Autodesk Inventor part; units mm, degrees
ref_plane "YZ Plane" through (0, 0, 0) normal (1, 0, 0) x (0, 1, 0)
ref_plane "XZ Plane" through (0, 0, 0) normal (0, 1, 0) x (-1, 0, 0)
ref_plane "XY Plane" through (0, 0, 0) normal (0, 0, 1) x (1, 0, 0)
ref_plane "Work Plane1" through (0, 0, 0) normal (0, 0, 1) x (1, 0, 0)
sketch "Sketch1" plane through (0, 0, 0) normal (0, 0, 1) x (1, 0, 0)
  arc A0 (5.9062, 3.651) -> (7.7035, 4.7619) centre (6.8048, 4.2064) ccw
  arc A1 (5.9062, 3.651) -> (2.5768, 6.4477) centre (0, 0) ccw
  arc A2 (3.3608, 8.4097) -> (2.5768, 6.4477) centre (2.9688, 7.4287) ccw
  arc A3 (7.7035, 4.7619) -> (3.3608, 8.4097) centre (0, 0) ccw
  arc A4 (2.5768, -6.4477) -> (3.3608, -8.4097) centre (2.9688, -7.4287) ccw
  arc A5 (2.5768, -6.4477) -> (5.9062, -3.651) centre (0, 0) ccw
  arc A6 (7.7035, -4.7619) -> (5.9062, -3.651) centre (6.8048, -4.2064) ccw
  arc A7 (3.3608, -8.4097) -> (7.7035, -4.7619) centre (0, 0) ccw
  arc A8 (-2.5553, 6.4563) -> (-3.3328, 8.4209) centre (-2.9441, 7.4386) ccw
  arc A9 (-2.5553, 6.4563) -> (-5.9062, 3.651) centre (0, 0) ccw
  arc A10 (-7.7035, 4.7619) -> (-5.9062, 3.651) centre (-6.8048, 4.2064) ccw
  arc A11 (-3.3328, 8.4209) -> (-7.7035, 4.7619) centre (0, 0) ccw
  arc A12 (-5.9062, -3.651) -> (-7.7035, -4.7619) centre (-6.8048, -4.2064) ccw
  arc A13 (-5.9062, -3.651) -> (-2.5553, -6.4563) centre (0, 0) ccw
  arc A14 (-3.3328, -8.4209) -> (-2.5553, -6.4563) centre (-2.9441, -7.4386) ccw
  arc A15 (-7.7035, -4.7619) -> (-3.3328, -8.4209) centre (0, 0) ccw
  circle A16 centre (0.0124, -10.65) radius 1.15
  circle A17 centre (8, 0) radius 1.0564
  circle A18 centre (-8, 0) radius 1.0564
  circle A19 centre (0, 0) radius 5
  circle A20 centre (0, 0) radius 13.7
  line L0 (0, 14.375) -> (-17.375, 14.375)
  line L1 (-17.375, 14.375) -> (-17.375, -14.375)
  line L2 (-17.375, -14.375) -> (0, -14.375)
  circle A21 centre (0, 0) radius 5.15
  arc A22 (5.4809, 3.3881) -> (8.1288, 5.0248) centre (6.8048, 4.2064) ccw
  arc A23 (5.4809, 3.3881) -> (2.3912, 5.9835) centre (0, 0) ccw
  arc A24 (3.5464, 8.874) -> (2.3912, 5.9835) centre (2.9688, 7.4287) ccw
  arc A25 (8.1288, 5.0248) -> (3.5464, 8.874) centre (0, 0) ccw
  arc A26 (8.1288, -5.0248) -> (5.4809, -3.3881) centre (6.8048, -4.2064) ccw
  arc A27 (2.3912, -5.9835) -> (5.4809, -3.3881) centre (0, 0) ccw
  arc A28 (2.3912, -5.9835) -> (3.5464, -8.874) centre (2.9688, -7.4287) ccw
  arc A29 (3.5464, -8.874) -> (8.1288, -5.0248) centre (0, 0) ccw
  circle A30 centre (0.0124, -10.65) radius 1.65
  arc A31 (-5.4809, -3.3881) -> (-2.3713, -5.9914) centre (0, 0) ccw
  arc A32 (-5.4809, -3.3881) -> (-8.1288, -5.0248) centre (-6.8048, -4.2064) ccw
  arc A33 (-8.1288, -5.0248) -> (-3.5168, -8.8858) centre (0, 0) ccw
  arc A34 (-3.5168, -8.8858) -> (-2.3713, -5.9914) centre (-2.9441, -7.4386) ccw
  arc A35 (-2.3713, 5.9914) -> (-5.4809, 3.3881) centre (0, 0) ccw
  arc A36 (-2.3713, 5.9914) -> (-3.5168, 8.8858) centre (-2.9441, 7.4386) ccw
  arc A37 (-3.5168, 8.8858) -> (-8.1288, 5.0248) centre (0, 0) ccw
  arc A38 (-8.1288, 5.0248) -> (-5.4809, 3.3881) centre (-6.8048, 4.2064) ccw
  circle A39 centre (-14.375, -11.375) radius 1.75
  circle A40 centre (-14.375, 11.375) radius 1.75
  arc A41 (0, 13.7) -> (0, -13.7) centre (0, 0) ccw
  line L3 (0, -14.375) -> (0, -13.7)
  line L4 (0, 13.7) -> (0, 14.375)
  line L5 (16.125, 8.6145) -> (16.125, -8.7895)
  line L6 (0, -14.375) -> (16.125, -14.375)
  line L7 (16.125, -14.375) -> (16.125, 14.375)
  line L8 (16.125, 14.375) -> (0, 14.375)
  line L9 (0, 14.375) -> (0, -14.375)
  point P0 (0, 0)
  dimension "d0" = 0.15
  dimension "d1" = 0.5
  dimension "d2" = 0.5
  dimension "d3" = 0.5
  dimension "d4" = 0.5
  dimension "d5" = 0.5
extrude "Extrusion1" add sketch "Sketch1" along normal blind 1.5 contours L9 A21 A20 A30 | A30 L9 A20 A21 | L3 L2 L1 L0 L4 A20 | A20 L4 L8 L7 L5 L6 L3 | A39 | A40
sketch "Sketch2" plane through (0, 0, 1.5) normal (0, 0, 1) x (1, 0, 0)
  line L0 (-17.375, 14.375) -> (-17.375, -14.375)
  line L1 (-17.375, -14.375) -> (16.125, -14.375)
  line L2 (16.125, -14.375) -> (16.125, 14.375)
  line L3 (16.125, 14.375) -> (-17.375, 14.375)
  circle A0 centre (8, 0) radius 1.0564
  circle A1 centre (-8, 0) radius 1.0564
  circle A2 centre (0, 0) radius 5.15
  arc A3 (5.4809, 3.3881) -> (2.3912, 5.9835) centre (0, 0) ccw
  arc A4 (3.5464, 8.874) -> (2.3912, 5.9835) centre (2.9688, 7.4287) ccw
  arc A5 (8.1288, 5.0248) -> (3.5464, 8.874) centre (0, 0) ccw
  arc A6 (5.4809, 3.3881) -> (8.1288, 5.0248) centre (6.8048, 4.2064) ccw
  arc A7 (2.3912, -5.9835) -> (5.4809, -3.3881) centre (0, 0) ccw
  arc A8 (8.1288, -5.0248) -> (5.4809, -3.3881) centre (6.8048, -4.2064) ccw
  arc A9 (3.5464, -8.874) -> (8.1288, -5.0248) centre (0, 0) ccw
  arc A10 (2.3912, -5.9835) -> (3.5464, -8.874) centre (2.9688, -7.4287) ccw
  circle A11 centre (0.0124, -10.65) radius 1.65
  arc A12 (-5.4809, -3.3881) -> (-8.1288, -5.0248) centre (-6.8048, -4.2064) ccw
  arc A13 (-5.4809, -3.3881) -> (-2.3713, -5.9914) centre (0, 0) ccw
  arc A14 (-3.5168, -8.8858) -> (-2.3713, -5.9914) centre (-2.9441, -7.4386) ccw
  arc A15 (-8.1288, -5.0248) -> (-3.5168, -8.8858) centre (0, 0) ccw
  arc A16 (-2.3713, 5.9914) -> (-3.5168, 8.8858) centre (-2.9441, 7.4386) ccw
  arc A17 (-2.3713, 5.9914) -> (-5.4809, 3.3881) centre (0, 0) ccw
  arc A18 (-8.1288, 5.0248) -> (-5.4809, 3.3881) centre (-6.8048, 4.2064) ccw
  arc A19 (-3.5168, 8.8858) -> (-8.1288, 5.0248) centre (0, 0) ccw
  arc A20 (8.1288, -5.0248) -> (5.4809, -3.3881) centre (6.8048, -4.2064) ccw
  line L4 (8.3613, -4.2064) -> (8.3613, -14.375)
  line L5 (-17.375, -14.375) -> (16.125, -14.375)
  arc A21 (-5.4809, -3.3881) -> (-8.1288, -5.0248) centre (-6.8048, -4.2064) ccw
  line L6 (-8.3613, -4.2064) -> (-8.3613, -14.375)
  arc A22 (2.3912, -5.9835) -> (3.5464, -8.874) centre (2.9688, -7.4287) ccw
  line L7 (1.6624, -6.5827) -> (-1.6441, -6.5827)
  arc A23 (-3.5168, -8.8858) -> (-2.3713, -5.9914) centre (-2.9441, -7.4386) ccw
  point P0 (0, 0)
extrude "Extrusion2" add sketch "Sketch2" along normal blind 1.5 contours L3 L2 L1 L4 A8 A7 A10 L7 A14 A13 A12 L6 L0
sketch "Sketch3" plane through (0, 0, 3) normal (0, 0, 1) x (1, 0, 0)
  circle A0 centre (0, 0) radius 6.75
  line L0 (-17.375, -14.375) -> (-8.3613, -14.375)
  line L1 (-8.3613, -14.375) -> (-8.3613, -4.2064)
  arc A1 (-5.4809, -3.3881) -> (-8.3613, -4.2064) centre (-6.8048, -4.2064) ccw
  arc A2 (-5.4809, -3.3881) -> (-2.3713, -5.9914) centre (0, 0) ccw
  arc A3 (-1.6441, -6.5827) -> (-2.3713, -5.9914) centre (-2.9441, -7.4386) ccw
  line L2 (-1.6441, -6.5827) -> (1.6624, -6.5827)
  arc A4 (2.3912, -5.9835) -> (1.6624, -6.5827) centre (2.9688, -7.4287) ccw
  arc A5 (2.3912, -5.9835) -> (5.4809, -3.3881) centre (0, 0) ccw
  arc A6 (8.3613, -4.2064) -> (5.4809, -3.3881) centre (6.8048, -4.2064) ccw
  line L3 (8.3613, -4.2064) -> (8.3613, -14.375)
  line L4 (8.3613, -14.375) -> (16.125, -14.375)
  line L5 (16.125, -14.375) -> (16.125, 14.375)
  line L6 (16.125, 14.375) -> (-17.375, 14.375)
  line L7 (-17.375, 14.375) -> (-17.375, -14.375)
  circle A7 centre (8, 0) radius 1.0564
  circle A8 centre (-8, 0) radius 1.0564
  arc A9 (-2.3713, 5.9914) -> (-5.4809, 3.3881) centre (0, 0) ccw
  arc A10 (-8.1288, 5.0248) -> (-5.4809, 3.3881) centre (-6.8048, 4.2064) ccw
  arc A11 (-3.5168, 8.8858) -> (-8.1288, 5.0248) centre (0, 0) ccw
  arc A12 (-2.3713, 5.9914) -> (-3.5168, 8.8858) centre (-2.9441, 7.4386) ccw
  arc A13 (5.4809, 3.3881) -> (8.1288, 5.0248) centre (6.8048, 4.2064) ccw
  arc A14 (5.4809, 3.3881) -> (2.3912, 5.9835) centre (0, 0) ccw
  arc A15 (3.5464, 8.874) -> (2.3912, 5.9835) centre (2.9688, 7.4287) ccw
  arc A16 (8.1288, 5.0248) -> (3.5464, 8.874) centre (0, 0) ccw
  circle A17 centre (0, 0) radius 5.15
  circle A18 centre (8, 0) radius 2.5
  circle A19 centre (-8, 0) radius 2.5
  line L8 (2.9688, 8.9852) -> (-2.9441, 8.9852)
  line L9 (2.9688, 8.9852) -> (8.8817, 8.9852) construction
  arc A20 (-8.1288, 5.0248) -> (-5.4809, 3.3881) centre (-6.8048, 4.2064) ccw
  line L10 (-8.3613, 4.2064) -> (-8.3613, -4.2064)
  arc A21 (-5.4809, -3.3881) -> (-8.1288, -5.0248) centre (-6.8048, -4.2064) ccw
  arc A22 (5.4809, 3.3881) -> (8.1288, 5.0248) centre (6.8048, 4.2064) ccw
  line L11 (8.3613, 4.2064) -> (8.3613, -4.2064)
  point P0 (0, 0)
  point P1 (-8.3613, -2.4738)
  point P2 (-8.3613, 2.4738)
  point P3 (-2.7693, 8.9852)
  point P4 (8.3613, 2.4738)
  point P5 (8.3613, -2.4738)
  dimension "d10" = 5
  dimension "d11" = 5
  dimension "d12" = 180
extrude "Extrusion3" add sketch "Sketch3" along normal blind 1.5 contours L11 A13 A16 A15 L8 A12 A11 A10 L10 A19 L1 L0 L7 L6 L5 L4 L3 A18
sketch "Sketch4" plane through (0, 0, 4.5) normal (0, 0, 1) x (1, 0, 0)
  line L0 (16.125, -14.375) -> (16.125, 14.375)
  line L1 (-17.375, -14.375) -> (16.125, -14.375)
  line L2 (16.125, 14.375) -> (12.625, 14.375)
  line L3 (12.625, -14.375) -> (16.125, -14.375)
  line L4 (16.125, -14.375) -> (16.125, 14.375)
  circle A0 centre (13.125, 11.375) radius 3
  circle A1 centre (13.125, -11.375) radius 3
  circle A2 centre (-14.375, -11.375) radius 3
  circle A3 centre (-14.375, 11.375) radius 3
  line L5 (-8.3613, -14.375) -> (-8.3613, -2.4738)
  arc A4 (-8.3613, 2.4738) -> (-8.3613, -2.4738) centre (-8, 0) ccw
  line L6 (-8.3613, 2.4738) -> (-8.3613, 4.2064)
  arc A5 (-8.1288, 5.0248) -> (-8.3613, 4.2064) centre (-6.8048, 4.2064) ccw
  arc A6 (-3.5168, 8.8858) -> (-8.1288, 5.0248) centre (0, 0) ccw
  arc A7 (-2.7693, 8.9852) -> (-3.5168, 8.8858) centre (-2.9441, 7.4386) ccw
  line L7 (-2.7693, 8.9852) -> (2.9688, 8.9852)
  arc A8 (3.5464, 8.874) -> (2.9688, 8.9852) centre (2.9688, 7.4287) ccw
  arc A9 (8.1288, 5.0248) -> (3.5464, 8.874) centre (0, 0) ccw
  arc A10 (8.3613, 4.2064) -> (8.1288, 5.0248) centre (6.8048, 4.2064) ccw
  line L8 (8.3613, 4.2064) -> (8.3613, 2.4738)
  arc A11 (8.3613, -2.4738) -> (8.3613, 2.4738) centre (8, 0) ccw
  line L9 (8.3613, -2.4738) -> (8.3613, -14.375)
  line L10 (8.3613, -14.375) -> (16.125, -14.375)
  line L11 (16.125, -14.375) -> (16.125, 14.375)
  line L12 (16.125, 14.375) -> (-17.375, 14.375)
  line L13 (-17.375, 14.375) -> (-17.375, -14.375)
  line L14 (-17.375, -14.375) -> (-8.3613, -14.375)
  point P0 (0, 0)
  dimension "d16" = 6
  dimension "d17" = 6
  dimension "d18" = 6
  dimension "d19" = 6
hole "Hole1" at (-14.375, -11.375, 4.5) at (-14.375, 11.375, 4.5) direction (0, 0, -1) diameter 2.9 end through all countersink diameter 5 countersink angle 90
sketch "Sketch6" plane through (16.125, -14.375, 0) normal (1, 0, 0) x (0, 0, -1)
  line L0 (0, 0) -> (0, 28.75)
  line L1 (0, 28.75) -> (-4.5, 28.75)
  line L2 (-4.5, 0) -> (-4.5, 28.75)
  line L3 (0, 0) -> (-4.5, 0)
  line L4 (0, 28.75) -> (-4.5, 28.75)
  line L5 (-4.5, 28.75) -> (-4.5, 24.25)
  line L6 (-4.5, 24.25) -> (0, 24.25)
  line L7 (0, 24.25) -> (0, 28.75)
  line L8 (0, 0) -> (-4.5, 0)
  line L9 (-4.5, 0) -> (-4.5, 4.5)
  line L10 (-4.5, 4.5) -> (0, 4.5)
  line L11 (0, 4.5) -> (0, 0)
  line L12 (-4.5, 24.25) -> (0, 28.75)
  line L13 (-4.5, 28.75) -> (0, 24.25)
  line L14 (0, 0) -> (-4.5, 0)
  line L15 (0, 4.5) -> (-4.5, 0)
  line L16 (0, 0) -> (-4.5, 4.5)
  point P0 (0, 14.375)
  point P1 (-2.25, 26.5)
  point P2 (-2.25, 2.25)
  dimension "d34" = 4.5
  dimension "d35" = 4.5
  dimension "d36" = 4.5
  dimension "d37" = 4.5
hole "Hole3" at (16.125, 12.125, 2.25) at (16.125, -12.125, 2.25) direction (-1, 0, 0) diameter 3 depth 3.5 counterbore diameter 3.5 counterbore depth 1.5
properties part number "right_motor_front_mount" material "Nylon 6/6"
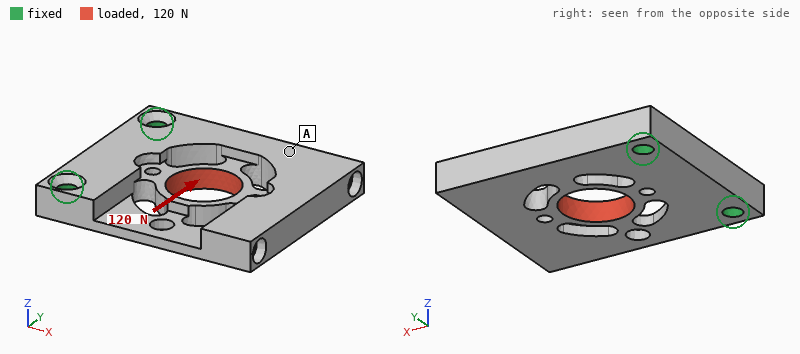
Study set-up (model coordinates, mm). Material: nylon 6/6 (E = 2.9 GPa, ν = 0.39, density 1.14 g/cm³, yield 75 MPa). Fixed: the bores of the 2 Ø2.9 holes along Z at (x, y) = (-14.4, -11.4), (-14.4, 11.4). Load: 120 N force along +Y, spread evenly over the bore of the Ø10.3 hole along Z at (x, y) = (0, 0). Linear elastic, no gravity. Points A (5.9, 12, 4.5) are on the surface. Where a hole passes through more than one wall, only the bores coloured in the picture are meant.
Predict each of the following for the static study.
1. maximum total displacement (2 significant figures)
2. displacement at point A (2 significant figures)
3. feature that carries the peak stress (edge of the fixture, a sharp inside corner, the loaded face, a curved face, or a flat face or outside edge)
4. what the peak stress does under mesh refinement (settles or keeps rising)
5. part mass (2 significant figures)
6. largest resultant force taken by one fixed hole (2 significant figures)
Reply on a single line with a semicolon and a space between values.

0.13 mm; 0.077 mm; a sharp inside corner; keeps rising; 3.3 g; 93 N
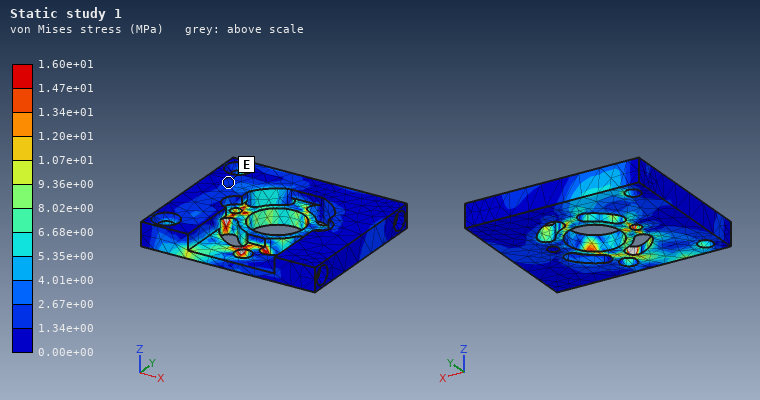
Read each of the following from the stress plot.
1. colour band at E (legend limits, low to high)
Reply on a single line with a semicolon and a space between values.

1.34e+00 to 2.67e+00 MPa
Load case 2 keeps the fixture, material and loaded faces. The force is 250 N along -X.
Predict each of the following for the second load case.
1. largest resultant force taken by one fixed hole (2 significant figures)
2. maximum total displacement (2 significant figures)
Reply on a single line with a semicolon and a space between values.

130 N; 0.14 mm
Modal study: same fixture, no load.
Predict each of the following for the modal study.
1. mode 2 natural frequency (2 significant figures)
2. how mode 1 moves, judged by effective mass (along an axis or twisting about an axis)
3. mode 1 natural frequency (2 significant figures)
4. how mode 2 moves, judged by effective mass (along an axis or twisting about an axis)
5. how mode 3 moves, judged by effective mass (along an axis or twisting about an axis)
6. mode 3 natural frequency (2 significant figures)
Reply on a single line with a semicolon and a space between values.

1800 Hz; along Z; 710 Hz; twisting about X; along Y; 3300 Hz
